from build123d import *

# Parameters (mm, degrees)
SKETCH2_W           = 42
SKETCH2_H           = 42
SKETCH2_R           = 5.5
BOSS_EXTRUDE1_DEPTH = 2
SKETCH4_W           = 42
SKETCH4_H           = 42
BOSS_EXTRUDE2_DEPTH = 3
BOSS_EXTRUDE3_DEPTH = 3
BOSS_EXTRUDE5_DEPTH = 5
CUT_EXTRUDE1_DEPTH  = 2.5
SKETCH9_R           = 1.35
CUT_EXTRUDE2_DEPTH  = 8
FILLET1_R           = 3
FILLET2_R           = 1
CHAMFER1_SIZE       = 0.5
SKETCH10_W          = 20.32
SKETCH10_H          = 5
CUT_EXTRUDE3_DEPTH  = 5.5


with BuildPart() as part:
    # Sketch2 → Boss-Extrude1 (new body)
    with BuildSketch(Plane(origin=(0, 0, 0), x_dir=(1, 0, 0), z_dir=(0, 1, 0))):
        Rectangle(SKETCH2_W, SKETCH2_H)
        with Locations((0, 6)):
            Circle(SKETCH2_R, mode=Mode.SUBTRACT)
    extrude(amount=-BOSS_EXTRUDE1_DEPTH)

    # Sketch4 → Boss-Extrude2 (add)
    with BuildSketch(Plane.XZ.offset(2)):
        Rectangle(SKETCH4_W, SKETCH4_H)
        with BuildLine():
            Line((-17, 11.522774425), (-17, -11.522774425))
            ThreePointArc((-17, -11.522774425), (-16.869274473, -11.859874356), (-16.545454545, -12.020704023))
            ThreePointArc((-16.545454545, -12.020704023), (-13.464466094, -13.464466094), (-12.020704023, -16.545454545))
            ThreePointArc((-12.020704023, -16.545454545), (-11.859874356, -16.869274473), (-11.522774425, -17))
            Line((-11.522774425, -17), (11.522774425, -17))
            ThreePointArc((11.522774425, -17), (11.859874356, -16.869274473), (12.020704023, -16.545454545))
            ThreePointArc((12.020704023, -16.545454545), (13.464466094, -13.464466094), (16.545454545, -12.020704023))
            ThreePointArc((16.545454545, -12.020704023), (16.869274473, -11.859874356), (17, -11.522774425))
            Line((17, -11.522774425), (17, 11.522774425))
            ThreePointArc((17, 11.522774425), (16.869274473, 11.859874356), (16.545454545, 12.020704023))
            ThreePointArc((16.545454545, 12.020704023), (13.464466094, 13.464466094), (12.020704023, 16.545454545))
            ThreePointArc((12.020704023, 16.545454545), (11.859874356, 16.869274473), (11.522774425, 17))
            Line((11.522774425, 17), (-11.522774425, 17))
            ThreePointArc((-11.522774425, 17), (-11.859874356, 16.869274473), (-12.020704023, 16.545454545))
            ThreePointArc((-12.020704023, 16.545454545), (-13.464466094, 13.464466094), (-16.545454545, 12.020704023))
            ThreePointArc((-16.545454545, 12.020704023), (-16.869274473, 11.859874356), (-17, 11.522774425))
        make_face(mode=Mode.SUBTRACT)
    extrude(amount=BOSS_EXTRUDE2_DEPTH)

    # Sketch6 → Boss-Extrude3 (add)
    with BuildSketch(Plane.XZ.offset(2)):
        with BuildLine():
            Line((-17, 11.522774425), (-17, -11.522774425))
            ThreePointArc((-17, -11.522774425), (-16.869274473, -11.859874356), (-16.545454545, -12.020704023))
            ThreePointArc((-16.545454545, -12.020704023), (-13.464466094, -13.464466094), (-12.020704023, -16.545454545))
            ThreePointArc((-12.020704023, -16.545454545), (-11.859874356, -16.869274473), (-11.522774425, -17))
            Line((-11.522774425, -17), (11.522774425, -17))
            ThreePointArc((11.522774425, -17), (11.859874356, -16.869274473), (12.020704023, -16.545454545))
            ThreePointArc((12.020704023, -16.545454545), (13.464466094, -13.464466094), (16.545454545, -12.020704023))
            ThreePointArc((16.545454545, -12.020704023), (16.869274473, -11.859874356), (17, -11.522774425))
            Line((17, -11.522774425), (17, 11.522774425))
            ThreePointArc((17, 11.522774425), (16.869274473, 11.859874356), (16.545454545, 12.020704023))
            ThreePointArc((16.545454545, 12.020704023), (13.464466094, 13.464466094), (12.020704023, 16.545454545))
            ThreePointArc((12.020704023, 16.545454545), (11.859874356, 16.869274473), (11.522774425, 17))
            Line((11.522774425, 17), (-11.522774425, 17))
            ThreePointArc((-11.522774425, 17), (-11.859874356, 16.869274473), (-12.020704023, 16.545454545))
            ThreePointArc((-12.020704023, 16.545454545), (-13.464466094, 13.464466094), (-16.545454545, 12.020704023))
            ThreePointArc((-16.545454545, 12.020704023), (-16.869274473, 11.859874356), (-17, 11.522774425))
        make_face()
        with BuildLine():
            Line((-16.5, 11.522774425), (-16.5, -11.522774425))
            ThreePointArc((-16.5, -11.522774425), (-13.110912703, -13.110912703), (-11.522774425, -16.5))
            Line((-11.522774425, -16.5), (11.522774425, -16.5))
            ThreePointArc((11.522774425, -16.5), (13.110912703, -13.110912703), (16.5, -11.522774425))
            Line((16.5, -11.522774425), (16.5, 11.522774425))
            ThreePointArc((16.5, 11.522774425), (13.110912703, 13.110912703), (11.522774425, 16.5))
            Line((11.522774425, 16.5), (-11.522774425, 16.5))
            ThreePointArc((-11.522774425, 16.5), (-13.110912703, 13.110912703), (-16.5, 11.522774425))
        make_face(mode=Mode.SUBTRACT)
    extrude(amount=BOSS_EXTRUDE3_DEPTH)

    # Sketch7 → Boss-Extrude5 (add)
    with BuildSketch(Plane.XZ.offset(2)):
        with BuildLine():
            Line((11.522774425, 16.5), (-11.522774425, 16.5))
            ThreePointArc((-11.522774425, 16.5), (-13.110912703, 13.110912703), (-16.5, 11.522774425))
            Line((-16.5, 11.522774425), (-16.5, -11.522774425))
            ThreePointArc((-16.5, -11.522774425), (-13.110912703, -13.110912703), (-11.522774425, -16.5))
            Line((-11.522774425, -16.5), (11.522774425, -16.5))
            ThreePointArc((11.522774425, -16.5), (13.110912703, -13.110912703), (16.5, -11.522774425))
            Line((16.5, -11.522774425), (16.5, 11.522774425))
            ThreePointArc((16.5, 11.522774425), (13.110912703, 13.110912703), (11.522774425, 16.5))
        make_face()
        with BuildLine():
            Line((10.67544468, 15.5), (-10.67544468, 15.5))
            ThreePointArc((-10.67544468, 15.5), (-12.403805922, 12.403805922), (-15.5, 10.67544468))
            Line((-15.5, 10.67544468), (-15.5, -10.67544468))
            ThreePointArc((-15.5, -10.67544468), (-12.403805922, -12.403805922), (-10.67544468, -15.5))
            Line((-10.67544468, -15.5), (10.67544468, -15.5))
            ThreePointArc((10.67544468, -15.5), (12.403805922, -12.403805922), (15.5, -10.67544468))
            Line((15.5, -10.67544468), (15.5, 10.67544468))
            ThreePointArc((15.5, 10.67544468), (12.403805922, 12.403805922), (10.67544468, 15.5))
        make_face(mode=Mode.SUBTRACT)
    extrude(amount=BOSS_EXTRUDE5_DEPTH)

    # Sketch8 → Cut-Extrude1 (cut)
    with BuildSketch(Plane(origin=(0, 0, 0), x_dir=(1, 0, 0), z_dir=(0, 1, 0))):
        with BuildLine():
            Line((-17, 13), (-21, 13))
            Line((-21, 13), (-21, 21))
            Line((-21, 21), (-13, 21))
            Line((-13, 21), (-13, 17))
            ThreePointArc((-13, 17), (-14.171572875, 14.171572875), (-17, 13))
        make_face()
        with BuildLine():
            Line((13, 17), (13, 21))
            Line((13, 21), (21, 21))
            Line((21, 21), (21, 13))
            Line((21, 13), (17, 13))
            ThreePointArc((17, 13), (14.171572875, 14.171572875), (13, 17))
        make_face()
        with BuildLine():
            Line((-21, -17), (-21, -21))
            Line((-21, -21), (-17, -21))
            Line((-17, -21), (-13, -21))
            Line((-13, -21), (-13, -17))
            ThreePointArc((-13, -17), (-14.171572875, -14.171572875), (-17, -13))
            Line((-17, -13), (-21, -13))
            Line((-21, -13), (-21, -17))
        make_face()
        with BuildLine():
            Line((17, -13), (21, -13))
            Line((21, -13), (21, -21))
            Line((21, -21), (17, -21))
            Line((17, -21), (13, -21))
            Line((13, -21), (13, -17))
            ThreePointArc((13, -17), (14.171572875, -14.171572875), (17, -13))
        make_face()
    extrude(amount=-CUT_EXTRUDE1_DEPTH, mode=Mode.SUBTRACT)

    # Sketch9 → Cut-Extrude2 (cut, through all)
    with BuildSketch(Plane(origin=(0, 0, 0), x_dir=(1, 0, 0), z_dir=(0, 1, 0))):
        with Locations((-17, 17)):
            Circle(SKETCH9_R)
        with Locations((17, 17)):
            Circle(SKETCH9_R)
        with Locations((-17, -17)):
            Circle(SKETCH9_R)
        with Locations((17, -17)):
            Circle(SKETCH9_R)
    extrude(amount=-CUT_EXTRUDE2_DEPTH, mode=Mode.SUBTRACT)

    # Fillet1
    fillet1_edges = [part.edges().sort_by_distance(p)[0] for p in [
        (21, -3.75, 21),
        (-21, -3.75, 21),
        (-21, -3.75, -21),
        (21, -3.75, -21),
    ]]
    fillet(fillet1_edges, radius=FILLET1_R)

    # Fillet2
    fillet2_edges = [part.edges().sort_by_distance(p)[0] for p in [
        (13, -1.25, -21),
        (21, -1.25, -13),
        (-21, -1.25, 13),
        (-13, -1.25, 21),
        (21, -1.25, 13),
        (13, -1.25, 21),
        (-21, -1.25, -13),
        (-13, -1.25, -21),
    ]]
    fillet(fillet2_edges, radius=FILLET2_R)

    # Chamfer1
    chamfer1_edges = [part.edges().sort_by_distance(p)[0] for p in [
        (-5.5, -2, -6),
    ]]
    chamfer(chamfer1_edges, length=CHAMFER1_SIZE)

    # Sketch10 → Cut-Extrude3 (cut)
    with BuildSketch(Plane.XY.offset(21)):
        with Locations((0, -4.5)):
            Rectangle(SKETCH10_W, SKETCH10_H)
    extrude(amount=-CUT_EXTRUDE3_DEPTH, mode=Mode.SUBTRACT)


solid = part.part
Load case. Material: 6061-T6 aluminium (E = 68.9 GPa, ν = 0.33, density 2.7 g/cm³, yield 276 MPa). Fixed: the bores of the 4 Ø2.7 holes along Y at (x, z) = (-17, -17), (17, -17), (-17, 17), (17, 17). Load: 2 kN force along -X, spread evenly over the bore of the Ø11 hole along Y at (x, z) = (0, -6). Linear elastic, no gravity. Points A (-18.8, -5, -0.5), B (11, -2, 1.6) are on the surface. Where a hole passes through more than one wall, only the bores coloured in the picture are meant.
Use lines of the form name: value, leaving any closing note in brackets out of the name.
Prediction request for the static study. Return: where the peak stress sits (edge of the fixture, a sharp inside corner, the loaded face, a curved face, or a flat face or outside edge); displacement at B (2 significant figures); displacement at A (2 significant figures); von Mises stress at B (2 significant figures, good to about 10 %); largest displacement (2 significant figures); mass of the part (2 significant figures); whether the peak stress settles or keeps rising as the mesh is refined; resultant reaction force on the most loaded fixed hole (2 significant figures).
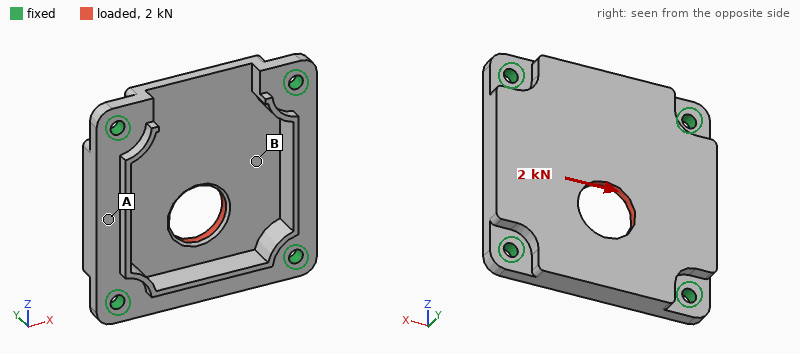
where the peak stress sits: edge of the fixture
displacement at B: 11 µm
displacement at A: 4.9 µm
von Mises stress at B: 23 MPa
largest displacement: 14 µm
mass of the part: 14 g
whether the peak stress settles or keeps rising as the mesh is refined: keeps rising
resultant reaction force on the most loaded fixed hole: 690 N
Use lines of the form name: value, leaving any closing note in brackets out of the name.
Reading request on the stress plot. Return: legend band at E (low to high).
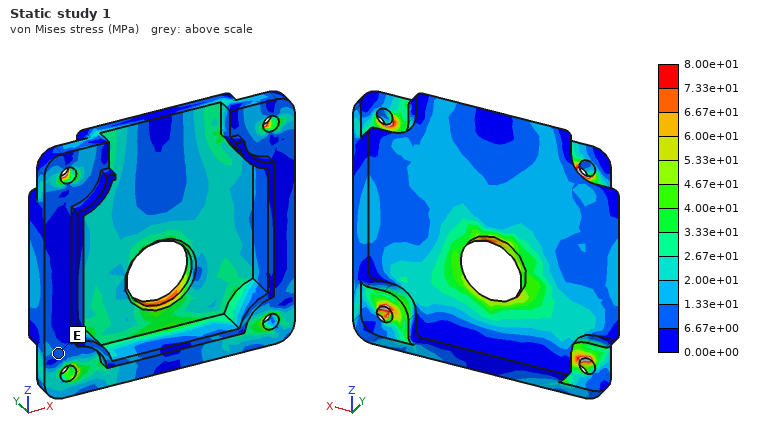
legend band at E: 6.67e+00 to 1.33e+01 MPa
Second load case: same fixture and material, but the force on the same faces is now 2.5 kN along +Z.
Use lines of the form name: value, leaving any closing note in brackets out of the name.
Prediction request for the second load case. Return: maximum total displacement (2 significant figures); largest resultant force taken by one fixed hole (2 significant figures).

maximum total displacement: 25 µm
largest resultant force taken by one fixed hole: 660 N
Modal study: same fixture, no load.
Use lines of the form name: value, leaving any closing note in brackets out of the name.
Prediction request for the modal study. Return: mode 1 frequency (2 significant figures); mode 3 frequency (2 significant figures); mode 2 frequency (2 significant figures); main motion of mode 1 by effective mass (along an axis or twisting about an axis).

mode 1 frequency: 11 kHz
mode 3 frequency: 16 kHz
mode 2 frequency: 16 kHz
main motion of mode 1 by effective mass: along Y
